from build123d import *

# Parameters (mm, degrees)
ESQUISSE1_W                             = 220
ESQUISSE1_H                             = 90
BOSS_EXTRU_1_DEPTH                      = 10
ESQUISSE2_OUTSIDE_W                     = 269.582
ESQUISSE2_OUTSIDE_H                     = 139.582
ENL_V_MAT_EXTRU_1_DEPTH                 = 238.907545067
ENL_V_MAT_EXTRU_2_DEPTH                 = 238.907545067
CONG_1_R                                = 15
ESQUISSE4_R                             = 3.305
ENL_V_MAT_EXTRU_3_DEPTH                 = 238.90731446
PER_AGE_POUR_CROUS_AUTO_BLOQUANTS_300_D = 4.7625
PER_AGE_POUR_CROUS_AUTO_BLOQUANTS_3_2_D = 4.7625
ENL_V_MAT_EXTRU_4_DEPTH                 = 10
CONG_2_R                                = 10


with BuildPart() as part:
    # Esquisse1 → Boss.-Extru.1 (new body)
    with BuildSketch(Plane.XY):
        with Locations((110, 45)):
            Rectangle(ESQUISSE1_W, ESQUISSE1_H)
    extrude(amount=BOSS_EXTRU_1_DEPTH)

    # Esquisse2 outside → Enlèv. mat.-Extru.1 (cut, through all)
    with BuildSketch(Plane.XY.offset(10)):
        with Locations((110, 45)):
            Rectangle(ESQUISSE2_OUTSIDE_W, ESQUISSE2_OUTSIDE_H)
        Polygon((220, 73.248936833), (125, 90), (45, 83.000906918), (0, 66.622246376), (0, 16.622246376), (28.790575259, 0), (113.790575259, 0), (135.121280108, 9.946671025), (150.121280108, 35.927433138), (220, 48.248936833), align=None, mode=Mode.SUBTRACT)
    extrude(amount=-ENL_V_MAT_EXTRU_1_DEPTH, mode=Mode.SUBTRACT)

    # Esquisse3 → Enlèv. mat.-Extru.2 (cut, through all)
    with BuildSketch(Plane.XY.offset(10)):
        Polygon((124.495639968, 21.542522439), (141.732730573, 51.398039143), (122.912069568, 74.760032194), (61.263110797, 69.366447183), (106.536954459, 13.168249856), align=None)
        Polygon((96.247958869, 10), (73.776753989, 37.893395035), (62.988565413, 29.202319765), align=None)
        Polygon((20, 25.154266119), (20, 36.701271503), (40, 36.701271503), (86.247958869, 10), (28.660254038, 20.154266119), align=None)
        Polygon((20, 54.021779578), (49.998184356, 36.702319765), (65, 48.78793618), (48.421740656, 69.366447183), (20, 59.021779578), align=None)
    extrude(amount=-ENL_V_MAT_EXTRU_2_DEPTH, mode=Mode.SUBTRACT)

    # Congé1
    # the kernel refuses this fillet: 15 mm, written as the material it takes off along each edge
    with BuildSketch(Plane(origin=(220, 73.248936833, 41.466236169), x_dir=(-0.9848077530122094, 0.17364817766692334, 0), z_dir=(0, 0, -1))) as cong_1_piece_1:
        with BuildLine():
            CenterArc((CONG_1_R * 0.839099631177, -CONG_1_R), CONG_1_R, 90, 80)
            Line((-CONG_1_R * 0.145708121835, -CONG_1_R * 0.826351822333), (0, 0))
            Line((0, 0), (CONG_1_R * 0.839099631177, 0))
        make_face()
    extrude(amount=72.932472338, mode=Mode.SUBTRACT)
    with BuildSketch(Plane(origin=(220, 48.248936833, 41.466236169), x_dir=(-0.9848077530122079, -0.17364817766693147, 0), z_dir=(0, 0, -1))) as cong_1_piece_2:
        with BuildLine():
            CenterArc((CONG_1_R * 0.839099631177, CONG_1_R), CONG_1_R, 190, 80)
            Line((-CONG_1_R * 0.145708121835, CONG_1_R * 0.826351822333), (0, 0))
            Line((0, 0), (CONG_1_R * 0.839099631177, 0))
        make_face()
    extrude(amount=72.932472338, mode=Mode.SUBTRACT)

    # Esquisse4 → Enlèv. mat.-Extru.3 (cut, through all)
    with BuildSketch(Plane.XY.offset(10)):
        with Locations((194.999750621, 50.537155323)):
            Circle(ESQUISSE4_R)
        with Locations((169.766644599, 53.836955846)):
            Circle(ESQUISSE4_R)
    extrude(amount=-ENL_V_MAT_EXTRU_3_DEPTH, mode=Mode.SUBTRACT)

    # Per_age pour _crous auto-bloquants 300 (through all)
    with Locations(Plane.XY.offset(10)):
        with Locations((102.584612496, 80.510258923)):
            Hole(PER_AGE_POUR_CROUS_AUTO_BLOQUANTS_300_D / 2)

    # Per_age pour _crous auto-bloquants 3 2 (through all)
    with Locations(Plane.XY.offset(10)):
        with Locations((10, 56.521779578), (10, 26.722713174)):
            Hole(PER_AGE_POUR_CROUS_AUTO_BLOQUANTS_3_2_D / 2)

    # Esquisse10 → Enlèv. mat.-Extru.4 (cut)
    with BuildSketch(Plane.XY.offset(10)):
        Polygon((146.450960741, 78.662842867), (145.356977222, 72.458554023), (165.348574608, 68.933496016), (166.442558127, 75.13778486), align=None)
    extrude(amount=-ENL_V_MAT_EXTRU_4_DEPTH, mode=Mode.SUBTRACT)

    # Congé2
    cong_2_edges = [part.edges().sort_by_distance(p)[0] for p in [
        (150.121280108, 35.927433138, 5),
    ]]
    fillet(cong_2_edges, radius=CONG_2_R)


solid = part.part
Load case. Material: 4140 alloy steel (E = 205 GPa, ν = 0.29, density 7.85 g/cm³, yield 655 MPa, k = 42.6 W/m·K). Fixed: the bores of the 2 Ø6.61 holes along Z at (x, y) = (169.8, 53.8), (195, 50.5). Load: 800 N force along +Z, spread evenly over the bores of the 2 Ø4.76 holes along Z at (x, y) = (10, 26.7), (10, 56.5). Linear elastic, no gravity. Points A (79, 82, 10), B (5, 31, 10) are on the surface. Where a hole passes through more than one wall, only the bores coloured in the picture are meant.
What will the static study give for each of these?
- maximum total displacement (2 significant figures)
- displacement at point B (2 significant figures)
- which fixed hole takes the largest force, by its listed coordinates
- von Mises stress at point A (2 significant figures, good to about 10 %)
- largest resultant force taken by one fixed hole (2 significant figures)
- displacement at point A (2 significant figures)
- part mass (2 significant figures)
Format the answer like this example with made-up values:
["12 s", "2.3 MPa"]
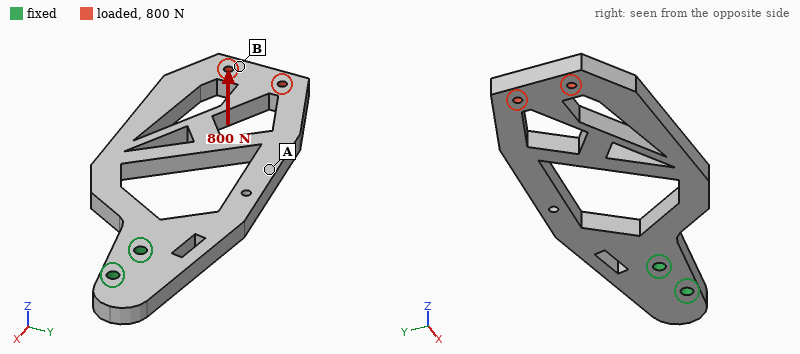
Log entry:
["2.3 mm", "2.2 mm", "(169.8, 53.8)", "110 MPa", "2.5 kN", "0.72 mm", "740 g"]
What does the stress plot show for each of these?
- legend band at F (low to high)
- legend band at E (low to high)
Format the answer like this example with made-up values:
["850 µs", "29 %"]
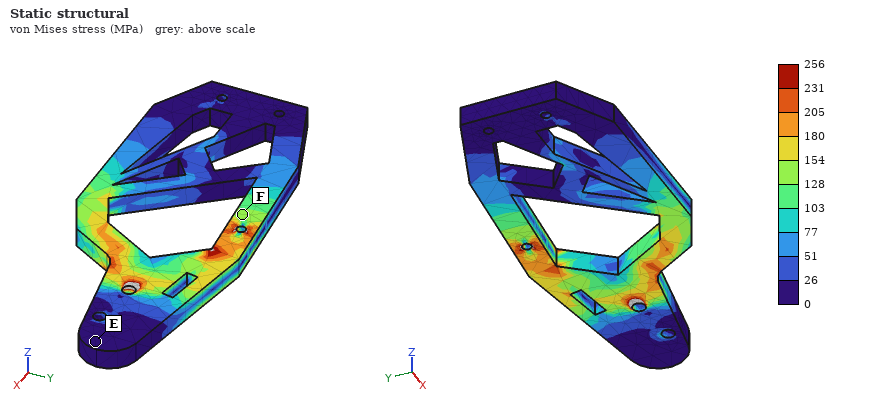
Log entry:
["128 to 154 MPa", "0 to 26 MPa"]
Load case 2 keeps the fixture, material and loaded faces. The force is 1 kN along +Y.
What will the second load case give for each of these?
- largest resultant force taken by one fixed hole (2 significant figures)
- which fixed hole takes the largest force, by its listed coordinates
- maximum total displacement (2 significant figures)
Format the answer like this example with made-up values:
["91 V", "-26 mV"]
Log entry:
["5.7 kN", "(169.8, 53.8)", "0.24 mm"]
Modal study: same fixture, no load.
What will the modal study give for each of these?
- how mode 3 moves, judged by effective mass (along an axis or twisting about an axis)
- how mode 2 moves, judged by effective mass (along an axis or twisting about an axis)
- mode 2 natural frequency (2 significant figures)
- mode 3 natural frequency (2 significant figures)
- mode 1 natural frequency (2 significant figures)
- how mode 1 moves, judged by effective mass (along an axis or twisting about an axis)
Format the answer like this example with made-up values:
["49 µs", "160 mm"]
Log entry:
["twisting about X", "along Y", "650 Hz", "780 Hz", "220 Hz", "along Z"]
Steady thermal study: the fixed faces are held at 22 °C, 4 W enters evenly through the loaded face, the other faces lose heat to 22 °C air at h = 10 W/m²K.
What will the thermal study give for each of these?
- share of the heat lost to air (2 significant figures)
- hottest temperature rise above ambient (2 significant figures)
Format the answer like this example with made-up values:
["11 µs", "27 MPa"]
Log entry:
["70 %", "22 K"]
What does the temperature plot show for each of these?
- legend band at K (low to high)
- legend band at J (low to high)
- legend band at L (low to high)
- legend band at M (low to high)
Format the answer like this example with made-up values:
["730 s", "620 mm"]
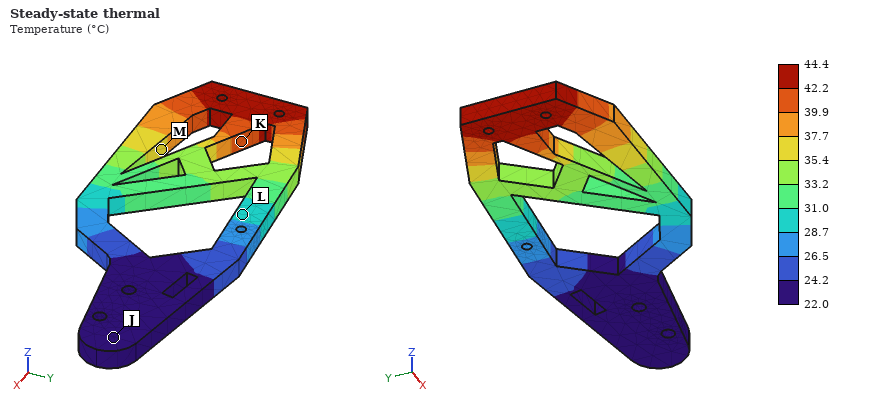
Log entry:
["39.9 to 42.2 °C", "22.0 to 24.2 °C", "28.7 to 31.0 °C", "35.4 to 37.7 °C"]
